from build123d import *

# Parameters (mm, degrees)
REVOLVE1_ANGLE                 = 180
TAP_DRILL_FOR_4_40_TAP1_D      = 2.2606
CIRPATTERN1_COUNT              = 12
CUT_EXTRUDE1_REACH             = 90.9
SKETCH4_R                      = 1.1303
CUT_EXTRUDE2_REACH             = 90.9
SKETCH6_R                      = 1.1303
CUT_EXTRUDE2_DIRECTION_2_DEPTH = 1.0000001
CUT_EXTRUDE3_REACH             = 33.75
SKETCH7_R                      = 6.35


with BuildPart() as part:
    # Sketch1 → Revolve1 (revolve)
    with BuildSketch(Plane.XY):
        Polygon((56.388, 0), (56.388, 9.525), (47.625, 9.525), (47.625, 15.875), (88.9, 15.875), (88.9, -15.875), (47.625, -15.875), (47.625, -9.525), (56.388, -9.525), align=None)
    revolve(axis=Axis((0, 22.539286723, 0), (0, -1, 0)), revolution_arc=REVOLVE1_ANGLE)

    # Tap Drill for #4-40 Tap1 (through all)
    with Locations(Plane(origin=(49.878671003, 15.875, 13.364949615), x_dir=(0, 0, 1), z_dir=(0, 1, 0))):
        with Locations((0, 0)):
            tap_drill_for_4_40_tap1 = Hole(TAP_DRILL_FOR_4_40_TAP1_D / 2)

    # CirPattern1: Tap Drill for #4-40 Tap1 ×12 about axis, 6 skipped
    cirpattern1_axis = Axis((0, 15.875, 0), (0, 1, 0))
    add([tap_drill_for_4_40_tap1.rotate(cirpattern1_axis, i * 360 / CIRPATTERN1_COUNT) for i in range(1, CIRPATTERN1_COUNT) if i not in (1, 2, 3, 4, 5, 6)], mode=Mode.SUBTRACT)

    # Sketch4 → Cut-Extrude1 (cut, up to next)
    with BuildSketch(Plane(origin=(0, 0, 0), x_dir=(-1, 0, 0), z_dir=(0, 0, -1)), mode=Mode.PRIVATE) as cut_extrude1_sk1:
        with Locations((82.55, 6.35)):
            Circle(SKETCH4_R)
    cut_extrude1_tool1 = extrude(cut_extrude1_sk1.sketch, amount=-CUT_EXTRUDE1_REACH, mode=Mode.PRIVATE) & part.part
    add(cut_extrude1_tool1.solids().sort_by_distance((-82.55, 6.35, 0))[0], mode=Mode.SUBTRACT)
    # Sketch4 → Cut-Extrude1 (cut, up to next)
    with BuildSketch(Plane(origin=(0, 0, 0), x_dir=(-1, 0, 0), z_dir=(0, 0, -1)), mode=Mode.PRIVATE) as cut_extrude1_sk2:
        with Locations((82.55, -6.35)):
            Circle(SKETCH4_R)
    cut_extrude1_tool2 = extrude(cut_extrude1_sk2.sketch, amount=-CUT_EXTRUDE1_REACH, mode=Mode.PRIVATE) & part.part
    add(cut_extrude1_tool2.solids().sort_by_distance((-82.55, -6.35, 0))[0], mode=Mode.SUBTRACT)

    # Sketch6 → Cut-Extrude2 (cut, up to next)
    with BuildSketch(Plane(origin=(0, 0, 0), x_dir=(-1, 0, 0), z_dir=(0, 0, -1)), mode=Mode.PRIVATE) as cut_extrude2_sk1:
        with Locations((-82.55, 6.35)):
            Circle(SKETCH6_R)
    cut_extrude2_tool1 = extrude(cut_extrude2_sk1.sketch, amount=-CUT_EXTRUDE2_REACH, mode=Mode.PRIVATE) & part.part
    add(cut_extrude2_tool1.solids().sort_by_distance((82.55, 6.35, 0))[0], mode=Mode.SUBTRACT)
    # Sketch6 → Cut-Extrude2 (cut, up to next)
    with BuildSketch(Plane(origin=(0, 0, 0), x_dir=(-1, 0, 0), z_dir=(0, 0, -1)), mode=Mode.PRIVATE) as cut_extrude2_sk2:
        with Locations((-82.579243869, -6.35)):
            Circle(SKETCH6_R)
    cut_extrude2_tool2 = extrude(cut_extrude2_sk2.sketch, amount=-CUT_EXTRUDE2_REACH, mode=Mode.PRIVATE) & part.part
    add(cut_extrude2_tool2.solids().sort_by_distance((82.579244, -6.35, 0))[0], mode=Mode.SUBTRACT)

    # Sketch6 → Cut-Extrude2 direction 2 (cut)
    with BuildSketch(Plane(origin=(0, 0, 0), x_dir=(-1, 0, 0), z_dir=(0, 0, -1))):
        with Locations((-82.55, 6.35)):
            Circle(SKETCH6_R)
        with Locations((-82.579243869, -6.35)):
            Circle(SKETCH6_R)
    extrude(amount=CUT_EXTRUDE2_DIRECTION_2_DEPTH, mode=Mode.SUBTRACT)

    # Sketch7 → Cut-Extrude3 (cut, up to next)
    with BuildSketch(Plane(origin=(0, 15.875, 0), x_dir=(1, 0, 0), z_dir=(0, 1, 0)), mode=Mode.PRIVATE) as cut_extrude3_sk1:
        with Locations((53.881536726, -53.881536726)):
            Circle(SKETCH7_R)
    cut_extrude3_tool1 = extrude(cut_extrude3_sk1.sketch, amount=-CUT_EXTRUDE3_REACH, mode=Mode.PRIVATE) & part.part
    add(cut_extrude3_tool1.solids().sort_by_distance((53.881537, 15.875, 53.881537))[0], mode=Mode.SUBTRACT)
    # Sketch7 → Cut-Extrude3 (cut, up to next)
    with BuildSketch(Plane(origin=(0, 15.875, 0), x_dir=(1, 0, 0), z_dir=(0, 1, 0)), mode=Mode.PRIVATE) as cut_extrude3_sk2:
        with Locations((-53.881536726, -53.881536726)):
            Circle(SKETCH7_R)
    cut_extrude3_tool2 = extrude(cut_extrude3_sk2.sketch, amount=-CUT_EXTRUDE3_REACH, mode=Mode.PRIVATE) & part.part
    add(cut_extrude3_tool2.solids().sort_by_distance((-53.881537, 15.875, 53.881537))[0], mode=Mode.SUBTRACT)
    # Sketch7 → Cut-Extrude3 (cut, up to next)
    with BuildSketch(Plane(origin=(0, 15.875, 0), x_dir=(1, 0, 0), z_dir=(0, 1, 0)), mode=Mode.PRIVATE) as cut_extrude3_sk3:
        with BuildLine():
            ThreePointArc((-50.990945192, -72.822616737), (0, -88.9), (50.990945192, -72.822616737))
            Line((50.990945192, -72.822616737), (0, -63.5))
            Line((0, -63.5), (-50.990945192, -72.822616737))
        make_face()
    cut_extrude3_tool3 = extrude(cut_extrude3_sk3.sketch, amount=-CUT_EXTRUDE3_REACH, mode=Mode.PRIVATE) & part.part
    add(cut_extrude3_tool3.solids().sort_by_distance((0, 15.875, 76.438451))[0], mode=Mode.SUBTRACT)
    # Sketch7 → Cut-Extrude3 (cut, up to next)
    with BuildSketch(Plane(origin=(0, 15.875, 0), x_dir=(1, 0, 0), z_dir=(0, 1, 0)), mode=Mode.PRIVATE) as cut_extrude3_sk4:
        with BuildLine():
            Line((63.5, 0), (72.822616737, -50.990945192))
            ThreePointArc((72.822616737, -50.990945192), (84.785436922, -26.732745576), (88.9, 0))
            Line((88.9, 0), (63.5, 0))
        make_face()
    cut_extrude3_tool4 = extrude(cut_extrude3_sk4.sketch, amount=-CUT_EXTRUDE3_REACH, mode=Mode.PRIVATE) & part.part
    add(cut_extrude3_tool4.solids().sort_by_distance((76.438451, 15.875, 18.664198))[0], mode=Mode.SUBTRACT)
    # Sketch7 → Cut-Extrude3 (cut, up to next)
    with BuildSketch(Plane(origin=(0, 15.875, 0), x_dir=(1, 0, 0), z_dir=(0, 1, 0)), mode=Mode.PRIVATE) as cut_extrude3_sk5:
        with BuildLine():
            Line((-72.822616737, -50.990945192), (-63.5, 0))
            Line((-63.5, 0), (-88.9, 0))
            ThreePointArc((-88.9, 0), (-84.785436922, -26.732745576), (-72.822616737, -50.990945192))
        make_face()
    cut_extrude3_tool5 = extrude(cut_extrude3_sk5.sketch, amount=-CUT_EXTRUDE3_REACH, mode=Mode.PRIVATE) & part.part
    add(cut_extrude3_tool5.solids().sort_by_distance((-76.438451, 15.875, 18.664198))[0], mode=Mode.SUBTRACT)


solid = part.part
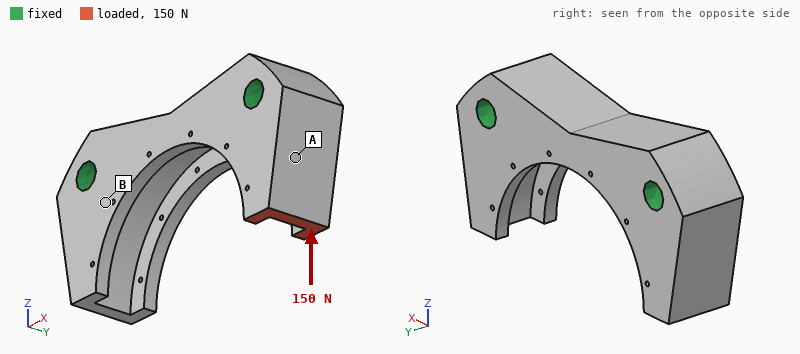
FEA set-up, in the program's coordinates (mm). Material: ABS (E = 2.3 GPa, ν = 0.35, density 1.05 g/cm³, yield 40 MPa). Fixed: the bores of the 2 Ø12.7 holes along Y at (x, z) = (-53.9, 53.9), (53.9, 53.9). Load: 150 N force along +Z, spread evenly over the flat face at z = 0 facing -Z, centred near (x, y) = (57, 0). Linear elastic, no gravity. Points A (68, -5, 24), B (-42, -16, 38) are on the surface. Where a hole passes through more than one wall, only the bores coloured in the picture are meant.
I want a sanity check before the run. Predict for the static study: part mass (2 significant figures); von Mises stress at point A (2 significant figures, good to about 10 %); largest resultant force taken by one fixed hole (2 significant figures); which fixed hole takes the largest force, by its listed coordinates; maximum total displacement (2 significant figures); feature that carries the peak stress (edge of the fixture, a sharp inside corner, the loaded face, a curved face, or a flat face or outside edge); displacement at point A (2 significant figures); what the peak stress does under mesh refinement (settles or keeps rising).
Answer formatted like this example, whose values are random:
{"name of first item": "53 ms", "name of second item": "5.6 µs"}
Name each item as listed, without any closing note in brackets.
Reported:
{"part mass": "150 g", "von Mises stress at point A": "0.23 MPa", "largest resultant force taken by one fixed hole": "150 N", "which fixed hole takes the largest force, by its listed coordinates": "(53.9, 53.9)", "maximum total displacement": "7.3 µm", "feature that carries the peak stress": "a sharp inside corner", "displacement at point A": "3.7 µm", "what the peak stress does under mesh refinement": "keeps rising"}
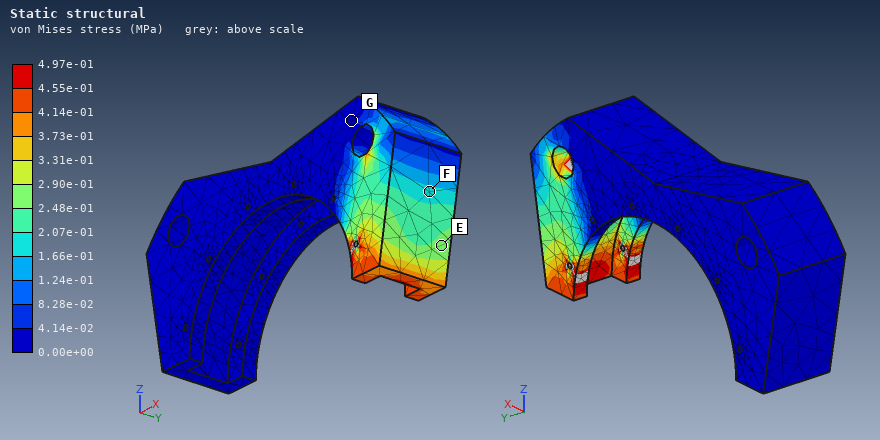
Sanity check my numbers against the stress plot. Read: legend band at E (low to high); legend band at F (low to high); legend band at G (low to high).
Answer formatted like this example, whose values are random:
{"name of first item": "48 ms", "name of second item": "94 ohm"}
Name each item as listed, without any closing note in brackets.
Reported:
{"legend band at E": "2.48e-01 to 2.90e-01 MPa", "legend band at F": "1.66e-01 to 2.07e-01 MPa", "legend band at G": "0.00e+00 to 4.14e-02 MPa"}
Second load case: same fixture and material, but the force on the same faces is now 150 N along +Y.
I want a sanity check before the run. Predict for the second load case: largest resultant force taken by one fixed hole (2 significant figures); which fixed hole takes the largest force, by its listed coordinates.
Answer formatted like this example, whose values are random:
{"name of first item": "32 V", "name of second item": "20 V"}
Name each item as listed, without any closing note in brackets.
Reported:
{"largest resultant force taken by one fixed hole": "150 N", "which fixed hole takes the largest force, by its listed coordinates": "(53.9, 53.9)"}
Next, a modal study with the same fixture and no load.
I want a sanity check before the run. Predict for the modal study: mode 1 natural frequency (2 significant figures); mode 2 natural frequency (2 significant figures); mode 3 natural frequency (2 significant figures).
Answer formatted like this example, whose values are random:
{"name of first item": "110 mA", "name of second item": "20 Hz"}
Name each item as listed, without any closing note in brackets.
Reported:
{"mode 1 natural frequency": "2300 Hz", "mode 2 natural frequency": "2800 Hz", "mode 3 natural frequency": "2900 Hz"}
